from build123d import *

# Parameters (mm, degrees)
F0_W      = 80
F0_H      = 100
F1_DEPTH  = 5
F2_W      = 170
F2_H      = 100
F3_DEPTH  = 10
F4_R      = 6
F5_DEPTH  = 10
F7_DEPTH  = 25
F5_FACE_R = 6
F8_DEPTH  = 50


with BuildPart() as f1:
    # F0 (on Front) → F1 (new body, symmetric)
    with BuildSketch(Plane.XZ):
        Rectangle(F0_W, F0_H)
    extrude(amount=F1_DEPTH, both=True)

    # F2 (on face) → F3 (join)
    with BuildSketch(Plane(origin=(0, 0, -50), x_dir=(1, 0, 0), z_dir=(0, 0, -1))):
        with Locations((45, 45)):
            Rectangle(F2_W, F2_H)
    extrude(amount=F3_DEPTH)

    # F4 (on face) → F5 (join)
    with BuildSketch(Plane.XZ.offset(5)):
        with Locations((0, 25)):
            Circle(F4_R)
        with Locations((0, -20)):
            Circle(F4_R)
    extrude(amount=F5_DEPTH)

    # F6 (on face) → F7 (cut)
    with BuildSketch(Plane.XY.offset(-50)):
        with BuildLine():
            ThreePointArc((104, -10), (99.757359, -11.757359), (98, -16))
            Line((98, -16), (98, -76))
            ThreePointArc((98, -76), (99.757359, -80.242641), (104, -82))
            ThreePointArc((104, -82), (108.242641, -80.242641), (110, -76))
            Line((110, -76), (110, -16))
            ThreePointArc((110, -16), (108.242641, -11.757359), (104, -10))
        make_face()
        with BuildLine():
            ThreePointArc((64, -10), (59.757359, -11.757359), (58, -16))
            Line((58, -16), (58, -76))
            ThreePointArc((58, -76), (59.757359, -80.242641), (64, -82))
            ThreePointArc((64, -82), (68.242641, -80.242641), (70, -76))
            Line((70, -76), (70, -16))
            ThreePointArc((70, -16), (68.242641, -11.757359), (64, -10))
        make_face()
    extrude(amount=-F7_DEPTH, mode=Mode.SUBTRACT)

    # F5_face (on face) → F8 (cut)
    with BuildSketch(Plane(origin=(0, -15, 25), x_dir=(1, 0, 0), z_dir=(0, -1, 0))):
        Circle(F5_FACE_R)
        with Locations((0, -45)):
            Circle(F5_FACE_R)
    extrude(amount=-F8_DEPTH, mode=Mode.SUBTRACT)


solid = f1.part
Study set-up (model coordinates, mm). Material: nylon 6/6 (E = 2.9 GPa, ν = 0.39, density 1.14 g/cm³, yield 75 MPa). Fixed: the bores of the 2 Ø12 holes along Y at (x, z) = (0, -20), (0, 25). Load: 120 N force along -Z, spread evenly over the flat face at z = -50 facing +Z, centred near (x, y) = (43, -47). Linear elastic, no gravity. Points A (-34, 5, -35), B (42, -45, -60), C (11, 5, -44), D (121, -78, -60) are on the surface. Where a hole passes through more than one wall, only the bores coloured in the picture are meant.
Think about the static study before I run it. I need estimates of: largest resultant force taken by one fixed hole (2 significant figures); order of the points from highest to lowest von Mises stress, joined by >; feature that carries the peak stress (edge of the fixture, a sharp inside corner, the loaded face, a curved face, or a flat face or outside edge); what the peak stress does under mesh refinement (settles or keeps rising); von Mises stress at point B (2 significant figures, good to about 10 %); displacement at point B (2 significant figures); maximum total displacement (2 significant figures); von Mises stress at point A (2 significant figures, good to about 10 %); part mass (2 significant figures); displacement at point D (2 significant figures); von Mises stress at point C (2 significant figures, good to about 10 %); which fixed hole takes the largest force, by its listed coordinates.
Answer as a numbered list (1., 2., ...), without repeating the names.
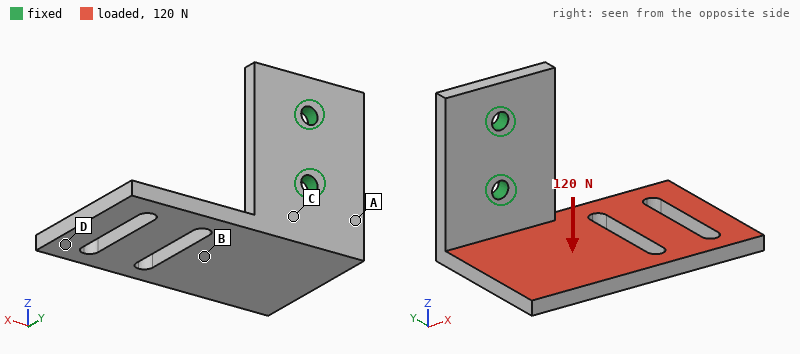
1. 130 N
2. C > A > B > D
3. edge of the fixture
4. keeps rising
5. 1.2 MPa
6. 0.78 mm
7. 2.7 mm
8. 3.1 MPa
9. 260 g
10. 2.2 mm
11. 4.1 MPa
12. (0, -20)
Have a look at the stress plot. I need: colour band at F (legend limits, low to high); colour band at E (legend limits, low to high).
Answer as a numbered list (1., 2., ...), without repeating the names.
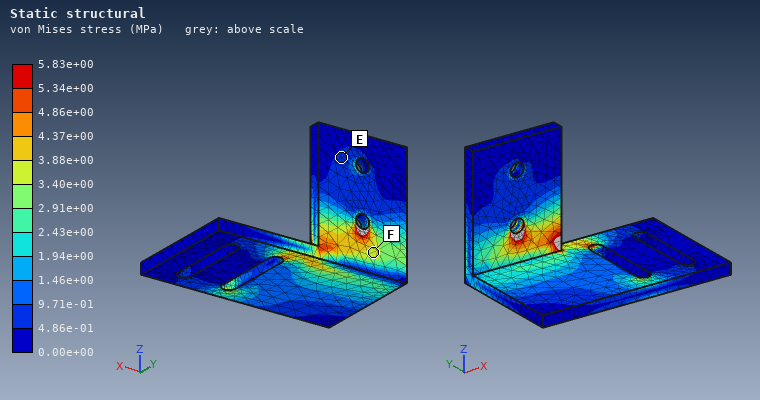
1. 3.40e+00 to 3.88e+00 MPa
2. 4.86e-01 to 9.71e-01 MPa
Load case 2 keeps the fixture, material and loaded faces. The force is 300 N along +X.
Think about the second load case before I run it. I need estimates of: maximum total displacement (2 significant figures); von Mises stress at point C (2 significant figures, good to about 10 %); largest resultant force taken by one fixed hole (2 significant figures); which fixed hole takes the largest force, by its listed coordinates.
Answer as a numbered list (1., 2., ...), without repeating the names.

1. 2.6 mm
2. 4.6 MPa
3. 440 N
4. (0, -20)
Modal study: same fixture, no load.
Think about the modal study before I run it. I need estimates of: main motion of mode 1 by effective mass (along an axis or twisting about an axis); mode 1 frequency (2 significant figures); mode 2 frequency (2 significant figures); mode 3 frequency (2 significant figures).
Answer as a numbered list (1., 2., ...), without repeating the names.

1. along Z
2. 110 Hz
3. 150 Hz
4. 200 Hz
